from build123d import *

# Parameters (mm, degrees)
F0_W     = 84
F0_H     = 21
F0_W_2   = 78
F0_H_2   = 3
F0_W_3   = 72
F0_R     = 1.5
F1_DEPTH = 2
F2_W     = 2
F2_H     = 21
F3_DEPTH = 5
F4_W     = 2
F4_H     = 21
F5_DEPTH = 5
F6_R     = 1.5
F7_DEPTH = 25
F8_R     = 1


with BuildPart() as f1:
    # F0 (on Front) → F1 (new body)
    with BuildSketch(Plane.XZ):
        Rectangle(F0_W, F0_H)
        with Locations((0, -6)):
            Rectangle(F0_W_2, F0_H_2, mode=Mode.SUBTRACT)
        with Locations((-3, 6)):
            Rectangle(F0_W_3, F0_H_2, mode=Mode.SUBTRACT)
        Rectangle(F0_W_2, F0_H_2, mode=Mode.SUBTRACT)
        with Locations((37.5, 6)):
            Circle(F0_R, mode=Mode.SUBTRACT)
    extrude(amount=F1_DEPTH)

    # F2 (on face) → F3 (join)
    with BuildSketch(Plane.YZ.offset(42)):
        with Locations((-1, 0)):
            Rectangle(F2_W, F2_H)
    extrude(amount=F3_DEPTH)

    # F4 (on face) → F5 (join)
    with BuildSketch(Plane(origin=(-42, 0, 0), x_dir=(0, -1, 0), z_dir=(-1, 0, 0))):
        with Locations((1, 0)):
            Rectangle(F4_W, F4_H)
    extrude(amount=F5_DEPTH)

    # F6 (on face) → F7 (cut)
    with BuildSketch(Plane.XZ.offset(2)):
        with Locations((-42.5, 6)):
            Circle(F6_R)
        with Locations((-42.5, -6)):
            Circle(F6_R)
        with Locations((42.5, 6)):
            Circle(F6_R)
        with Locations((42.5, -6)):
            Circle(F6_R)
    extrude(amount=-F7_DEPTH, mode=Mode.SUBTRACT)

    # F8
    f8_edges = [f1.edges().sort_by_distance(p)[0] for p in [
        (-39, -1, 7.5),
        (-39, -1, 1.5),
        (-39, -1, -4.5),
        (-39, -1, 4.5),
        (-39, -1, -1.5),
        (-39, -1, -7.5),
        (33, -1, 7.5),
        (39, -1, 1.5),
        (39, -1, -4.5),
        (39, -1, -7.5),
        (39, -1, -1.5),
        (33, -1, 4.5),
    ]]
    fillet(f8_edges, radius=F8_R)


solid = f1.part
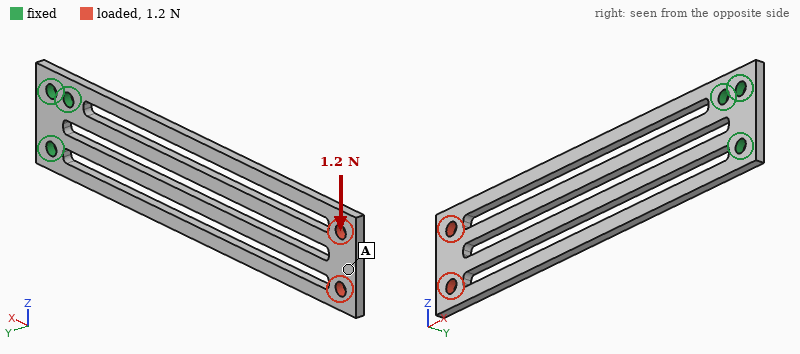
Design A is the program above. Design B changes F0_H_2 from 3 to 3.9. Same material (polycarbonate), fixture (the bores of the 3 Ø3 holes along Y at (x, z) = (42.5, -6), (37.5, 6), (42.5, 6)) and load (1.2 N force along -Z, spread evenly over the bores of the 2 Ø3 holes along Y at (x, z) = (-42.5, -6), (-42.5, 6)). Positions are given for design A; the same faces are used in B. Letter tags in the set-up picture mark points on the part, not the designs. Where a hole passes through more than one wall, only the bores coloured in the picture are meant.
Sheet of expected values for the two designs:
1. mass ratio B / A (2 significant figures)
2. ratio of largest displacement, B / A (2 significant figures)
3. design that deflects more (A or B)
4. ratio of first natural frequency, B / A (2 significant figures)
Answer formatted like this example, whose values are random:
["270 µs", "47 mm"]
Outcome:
["0.84", "2.0", "B", "0.95"]
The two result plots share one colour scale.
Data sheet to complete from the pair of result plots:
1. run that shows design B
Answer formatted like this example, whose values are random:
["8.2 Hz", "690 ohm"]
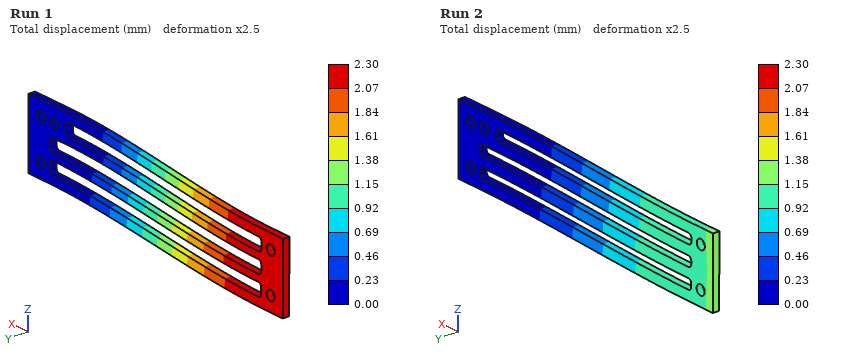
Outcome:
["Run 1"]
